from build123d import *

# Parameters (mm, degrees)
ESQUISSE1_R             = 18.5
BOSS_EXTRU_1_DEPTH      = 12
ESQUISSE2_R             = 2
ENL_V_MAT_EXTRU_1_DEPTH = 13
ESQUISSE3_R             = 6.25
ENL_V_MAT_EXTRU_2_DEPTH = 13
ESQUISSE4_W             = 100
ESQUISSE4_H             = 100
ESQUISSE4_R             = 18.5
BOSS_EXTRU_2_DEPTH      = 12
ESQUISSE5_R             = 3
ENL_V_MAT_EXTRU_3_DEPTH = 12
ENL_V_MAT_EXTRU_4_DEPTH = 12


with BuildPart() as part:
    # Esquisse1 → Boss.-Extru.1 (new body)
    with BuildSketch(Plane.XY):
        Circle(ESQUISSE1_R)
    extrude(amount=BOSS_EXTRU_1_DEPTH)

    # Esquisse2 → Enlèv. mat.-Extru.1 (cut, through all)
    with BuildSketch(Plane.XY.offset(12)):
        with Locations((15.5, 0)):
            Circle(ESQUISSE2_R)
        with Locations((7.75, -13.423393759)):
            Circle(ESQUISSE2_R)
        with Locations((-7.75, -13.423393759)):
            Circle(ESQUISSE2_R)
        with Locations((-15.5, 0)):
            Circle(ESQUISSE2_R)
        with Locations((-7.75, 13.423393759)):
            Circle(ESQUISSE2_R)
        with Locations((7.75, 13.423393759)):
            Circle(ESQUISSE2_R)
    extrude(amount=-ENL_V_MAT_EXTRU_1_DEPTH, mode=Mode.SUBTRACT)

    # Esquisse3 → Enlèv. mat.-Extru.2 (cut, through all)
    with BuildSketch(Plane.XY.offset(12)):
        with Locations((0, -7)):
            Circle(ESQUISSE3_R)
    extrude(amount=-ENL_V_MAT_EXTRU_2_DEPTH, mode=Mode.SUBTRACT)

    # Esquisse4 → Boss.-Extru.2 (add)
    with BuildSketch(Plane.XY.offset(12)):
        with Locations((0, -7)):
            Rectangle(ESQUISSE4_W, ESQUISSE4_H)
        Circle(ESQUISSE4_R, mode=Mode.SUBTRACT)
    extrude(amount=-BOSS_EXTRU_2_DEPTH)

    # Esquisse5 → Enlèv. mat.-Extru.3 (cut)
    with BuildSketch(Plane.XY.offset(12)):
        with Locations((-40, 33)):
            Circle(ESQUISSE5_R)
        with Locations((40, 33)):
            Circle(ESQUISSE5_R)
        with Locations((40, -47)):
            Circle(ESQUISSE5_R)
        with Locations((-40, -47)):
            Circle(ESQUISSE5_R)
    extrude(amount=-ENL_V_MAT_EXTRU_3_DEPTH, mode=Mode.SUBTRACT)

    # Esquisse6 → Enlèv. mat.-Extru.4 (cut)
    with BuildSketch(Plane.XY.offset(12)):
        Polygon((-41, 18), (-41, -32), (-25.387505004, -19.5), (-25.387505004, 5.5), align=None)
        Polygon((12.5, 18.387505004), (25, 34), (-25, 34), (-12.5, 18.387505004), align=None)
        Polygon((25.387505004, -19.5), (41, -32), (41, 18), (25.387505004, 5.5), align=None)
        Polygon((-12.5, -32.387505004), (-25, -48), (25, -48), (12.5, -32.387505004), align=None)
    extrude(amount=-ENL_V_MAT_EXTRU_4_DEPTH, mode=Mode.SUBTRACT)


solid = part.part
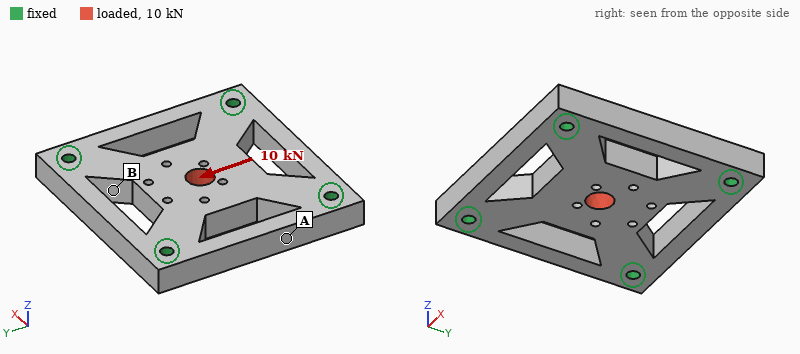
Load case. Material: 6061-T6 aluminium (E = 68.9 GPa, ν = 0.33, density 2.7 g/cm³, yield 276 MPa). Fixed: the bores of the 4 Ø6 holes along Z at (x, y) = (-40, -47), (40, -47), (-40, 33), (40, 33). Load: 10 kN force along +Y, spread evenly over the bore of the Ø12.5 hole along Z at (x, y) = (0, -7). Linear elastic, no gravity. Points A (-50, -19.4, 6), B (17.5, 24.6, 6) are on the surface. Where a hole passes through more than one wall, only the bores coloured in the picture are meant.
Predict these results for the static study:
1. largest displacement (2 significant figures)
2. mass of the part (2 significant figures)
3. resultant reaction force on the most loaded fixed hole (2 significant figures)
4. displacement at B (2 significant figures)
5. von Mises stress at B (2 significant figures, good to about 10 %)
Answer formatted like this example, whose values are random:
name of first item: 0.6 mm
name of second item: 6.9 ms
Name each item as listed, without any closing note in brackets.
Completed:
largest displacement: 16 µm
mass of the part: 240 g
resultant reaction force on the most loaded fixed hole: 3.1 kN
displacement at B: 7.9 µm
von Mises stress at B: 14 MPa
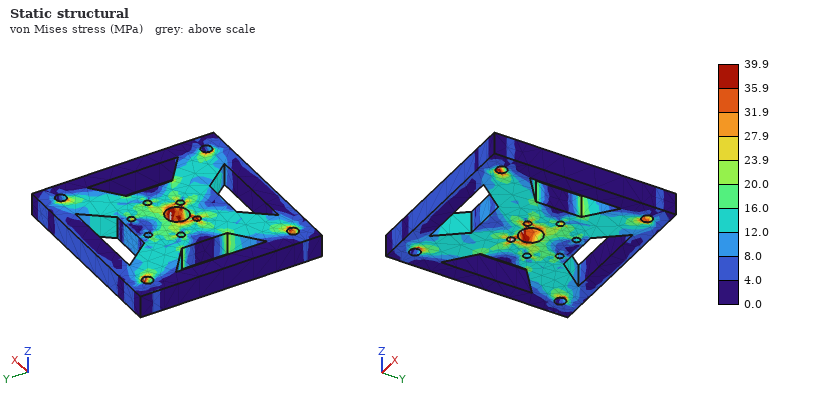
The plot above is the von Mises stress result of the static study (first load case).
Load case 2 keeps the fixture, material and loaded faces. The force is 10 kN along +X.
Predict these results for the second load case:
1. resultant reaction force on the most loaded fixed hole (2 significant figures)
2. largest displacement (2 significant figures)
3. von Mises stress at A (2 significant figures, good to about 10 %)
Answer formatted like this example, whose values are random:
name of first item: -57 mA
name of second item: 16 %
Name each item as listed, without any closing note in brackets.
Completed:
resultant reaction force on the most loaded fixed hole: 3.1 kN
largest displacement: 17 µm
von Mises stress at A: 4.3 MPa
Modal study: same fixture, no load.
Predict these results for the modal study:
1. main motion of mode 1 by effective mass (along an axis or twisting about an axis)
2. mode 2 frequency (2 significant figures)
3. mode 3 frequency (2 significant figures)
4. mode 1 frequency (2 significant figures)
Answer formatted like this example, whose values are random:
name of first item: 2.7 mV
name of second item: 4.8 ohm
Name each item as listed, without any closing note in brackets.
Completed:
main motion of mode 1 by effective mass: along Z
mode 2 frequency: 9700 Hz
mode 3 frequency: 9700 Hz
mode 1 frequency: 5600 Hz
